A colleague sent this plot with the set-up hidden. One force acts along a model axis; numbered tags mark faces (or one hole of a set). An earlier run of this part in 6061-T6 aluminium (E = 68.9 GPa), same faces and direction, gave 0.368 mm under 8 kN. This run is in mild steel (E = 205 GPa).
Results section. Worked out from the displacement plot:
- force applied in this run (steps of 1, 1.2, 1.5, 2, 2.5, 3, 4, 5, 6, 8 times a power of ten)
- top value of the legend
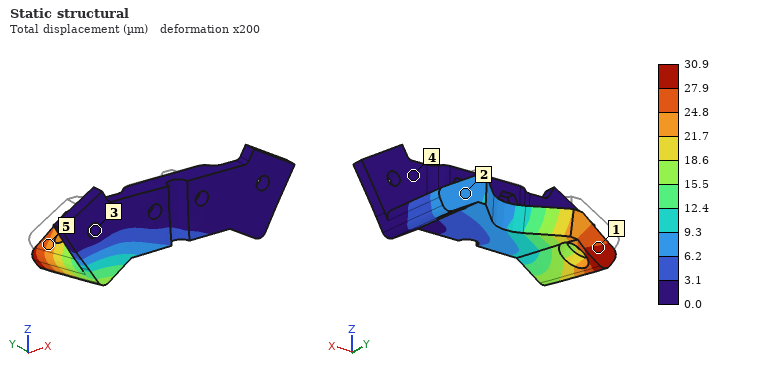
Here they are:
2 kN
30.9 µm
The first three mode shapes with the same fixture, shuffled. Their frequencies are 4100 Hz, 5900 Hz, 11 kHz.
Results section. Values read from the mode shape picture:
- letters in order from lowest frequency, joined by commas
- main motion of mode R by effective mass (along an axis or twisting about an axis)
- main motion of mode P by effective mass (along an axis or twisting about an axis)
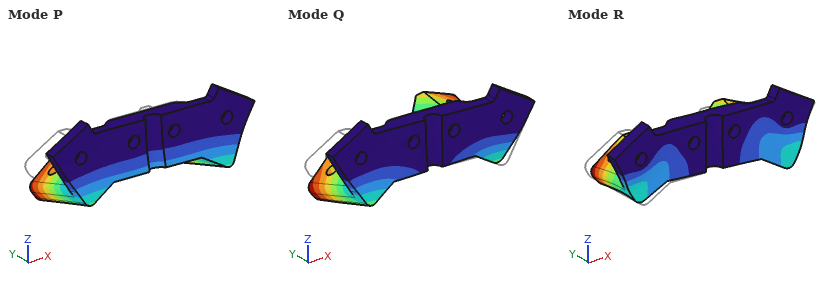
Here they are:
P, Q, R
along X
along Z
